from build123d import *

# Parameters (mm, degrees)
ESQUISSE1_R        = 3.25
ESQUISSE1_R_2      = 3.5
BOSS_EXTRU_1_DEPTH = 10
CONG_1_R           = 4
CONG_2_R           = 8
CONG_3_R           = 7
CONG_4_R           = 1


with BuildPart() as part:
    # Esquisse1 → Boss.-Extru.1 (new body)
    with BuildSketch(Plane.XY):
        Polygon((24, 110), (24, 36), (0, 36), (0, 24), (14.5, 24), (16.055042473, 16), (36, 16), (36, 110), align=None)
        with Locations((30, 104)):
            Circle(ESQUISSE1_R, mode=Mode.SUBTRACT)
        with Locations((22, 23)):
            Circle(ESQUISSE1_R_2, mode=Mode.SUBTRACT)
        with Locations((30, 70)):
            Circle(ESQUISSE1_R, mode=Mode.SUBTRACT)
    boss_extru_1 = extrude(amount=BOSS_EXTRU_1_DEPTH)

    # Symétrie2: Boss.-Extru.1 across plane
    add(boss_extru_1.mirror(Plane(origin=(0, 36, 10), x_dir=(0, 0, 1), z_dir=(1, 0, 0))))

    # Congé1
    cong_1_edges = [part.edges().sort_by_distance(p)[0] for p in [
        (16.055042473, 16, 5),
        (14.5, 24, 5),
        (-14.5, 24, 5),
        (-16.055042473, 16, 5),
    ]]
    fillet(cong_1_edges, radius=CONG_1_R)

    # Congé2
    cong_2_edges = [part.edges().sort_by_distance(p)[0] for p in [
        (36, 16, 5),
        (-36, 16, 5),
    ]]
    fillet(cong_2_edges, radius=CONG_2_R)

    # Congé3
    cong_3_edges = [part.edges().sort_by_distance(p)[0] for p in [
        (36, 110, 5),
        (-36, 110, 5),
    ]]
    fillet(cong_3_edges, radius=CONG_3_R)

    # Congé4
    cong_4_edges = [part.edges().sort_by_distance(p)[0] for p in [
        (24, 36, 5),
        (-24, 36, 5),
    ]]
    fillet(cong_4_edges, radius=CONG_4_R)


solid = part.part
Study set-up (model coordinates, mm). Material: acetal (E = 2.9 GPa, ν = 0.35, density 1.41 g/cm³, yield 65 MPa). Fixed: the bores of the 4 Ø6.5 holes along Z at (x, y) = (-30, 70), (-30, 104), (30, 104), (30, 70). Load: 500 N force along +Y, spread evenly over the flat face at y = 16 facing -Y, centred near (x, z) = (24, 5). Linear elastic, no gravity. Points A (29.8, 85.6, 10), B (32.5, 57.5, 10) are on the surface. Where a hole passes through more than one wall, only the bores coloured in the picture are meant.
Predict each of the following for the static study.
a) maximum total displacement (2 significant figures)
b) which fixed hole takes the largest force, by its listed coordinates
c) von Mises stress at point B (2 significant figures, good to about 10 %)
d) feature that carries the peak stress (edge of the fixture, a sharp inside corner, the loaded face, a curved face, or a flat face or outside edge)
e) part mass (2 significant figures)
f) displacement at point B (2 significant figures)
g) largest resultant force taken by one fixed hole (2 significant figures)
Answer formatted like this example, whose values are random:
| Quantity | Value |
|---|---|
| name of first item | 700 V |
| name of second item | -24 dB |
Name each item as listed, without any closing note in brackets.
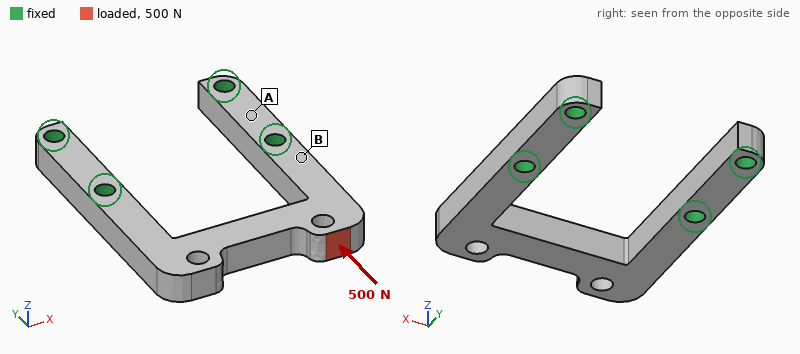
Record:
| Quantity | Value |
|---|---|
| maximum total displacement | 0.12 mm |
| which fixed hole takes the largest force, by its listed coordinates | (30, 70) |
| von Mises stress at point B | 3.7 MPa |
| feature that carries the peak stress | a curved face |
| part mass | 38 g |
| displacement at point B | 0.017 mm |
| largest resultant force taken by one fixed hole | 440 N |
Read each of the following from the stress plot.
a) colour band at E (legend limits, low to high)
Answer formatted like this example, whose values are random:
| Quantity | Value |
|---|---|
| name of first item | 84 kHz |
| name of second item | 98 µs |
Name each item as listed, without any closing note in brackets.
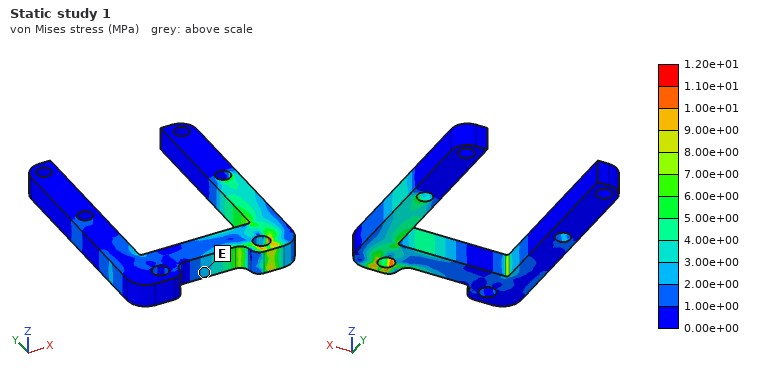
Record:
| Quantity | Value |
|---|---|
| colour band at E | 2.00e+00 to 3.00e+00 MPa |
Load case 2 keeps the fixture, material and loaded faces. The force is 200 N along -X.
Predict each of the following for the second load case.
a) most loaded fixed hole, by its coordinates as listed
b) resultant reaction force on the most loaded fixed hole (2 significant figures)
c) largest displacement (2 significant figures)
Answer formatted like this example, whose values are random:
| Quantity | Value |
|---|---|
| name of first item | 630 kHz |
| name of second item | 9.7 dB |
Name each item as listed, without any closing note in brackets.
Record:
| Quantity | Value |
|---|---|
| most loaded fixed hole, by its coordinates as listed | (-30, 70) |
| resultant reaction force on the most loaded fixed hole | 170 N |
| largest displacement | 0.32 mm |
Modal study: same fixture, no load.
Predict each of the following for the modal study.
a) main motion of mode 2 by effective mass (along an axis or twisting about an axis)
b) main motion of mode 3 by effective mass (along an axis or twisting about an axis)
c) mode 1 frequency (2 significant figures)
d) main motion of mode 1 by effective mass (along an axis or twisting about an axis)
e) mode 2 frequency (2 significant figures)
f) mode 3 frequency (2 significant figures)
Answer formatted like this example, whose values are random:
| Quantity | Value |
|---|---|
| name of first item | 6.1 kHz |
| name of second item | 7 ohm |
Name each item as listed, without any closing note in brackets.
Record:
| Quantity | Value |
|---|---|
| main motion of mode 2 by effective mass | twisting about Y |
| main motion of mode 3 by effective mass | along X |
| mode 1 frequency | 600 Hz |
| main motion of mode 1 by effective mass | along Z |
| mode 2 frequency | 1100 Hz |
| mode 3 frequency | 1200 Hz |
